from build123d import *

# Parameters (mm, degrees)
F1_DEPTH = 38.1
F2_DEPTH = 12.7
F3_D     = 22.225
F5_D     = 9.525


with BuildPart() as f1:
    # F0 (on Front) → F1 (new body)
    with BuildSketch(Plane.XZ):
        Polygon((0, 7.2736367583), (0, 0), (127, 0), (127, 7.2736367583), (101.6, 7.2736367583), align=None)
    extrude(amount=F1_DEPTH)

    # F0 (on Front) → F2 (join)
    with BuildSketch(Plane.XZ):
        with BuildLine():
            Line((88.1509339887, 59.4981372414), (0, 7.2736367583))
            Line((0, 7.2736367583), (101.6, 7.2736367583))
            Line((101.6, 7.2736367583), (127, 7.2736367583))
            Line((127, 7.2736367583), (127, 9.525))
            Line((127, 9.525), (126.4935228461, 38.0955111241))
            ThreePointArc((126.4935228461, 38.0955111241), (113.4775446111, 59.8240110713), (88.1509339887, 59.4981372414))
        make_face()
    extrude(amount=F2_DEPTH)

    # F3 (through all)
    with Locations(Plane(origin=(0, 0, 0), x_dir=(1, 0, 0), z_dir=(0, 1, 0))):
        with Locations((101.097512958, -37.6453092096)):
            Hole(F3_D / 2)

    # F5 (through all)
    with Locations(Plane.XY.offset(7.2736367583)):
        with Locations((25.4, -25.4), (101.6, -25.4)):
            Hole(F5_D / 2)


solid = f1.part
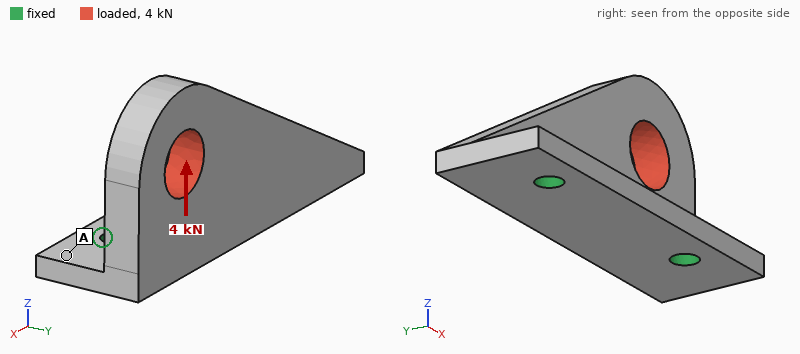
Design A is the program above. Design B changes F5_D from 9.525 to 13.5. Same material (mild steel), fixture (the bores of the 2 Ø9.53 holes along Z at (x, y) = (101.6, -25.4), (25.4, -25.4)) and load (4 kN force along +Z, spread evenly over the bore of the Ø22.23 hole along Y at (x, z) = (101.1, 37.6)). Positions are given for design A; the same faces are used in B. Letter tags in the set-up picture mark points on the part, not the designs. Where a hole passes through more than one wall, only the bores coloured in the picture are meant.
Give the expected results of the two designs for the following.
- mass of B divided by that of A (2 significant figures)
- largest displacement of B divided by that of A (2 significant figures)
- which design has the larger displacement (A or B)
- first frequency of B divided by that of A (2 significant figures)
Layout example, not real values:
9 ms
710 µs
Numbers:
0.99
0.73
A
1.1
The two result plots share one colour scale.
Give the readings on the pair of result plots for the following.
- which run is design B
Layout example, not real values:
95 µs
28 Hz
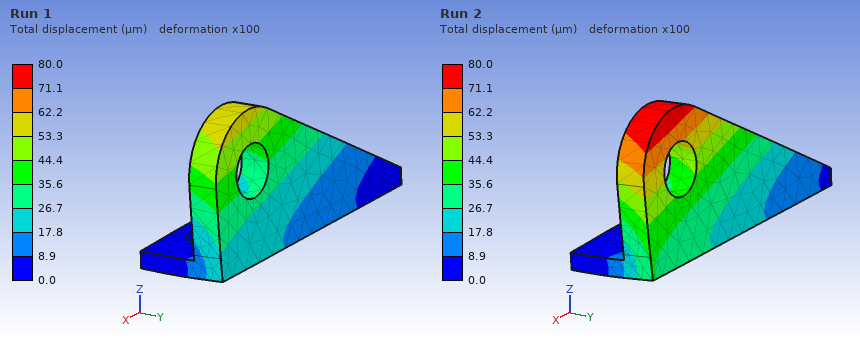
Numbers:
Run 1
